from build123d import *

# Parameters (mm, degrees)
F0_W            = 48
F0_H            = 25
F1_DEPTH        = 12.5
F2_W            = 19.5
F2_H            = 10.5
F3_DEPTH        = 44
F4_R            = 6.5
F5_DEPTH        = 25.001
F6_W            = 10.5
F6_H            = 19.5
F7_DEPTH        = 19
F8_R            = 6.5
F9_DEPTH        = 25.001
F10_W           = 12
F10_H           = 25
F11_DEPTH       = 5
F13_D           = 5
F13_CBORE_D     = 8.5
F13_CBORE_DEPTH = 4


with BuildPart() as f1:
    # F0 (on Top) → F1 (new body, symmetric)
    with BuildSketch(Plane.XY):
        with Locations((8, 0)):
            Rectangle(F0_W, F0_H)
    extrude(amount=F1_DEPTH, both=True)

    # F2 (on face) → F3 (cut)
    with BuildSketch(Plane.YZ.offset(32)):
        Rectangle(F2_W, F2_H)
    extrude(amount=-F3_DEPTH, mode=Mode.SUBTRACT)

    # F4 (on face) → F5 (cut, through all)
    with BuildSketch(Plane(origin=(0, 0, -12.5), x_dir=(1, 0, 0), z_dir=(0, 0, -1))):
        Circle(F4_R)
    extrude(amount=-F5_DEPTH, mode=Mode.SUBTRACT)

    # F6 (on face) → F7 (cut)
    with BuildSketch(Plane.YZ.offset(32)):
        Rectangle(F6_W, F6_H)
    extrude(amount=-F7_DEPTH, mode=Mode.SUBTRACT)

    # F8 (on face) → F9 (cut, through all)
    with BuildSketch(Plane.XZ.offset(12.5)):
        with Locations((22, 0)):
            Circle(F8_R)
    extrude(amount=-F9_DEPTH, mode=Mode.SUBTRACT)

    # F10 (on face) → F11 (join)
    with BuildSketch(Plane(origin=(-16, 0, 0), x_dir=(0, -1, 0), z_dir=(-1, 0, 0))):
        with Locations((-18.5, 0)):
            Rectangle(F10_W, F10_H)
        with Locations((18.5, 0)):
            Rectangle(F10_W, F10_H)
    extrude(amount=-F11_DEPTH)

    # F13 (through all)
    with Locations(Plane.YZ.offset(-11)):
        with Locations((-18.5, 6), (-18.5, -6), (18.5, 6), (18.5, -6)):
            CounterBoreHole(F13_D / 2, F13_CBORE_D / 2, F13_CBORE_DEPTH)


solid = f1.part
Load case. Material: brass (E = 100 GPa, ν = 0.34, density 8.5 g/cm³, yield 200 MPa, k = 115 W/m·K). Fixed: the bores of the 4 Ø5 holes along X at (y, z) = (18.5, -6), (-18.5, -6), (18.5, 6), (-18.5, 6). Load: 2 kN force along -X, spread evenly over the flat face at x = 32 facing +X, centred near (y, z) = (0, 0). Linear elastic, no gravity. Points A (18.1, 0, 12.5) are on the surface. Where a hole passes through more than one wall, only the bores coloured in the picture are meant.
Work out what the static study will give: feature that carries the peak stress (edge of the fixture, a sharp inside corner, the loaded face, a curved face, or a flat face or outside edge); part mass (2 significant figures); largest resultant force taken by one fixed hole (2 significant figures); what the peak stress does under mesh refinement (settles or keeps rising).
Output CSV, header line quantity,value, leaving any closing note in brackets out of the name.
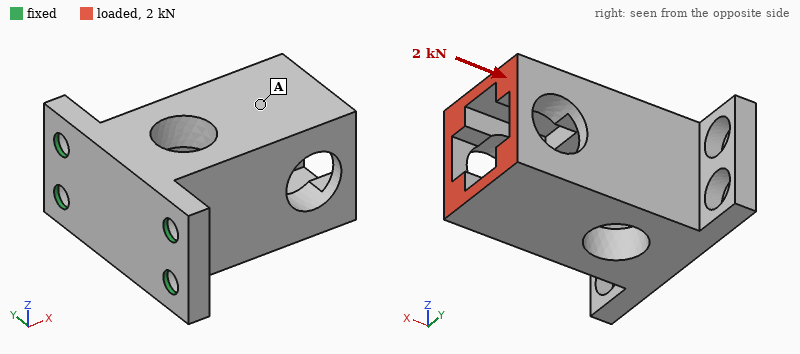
quantity,value
feature that carries the peak stress,edge of the fixture
part mass,160 g
largest resultant force taken by one fixed hole,650 N
what the peak stress does under mesh refinement,keeps rising
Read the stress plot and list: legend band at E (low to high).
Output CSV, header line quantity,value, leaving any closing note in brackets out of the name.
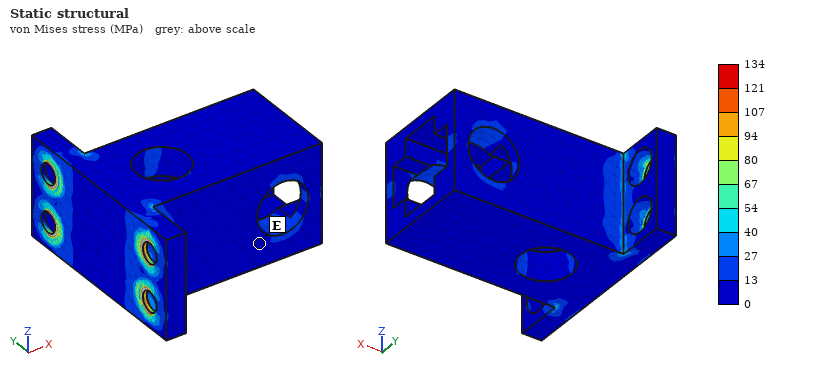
quantity,value
legend band at E,0 to 13 MPa
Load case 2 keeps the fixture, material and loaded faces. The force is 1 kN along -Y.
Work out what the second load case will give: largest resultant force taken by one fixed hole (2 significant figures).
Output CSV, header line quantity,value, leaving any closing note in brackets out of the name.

quantity,value
largest resultant force taken by one fixed hole,740 N
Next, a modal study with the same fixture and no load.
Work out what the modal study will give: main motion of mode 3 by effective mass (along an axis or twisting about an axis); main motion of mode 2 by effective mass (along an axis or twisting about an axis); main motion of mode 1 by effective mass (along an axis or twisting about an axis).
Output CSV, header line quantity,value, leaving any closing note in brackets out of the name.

quantity,value
main motion of mode 3 by effective mass,along X
main motion of mode 2 by effective mass,along Y
main motion of mode 1 by effective mass,along Z
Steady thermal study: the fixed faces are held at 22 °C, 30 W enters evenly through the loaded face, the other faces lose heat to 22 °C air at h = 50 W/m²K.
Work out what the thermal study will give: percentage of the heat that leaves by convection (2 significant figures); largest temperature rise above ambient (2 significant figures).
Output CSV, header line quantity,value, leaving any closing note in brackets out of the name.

quantity,value
percentage of the heat that leaves by convection,35 %
largest temperature rise above ambient,47 K
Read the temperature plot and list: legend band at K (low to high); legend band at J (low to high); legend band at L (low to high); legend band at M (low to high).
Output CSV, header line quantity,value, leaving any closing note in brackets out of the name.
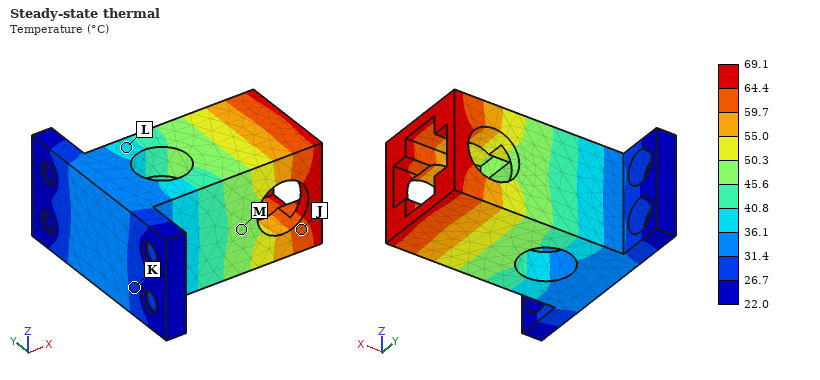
quantity,value
legend band at K,26.7 to 31.4 °C
legend band at J,59.7 to 64.4 °C
legend band at L,36.1 to 40.8 °C
legend band at M,45.6 to 50.3 °C
